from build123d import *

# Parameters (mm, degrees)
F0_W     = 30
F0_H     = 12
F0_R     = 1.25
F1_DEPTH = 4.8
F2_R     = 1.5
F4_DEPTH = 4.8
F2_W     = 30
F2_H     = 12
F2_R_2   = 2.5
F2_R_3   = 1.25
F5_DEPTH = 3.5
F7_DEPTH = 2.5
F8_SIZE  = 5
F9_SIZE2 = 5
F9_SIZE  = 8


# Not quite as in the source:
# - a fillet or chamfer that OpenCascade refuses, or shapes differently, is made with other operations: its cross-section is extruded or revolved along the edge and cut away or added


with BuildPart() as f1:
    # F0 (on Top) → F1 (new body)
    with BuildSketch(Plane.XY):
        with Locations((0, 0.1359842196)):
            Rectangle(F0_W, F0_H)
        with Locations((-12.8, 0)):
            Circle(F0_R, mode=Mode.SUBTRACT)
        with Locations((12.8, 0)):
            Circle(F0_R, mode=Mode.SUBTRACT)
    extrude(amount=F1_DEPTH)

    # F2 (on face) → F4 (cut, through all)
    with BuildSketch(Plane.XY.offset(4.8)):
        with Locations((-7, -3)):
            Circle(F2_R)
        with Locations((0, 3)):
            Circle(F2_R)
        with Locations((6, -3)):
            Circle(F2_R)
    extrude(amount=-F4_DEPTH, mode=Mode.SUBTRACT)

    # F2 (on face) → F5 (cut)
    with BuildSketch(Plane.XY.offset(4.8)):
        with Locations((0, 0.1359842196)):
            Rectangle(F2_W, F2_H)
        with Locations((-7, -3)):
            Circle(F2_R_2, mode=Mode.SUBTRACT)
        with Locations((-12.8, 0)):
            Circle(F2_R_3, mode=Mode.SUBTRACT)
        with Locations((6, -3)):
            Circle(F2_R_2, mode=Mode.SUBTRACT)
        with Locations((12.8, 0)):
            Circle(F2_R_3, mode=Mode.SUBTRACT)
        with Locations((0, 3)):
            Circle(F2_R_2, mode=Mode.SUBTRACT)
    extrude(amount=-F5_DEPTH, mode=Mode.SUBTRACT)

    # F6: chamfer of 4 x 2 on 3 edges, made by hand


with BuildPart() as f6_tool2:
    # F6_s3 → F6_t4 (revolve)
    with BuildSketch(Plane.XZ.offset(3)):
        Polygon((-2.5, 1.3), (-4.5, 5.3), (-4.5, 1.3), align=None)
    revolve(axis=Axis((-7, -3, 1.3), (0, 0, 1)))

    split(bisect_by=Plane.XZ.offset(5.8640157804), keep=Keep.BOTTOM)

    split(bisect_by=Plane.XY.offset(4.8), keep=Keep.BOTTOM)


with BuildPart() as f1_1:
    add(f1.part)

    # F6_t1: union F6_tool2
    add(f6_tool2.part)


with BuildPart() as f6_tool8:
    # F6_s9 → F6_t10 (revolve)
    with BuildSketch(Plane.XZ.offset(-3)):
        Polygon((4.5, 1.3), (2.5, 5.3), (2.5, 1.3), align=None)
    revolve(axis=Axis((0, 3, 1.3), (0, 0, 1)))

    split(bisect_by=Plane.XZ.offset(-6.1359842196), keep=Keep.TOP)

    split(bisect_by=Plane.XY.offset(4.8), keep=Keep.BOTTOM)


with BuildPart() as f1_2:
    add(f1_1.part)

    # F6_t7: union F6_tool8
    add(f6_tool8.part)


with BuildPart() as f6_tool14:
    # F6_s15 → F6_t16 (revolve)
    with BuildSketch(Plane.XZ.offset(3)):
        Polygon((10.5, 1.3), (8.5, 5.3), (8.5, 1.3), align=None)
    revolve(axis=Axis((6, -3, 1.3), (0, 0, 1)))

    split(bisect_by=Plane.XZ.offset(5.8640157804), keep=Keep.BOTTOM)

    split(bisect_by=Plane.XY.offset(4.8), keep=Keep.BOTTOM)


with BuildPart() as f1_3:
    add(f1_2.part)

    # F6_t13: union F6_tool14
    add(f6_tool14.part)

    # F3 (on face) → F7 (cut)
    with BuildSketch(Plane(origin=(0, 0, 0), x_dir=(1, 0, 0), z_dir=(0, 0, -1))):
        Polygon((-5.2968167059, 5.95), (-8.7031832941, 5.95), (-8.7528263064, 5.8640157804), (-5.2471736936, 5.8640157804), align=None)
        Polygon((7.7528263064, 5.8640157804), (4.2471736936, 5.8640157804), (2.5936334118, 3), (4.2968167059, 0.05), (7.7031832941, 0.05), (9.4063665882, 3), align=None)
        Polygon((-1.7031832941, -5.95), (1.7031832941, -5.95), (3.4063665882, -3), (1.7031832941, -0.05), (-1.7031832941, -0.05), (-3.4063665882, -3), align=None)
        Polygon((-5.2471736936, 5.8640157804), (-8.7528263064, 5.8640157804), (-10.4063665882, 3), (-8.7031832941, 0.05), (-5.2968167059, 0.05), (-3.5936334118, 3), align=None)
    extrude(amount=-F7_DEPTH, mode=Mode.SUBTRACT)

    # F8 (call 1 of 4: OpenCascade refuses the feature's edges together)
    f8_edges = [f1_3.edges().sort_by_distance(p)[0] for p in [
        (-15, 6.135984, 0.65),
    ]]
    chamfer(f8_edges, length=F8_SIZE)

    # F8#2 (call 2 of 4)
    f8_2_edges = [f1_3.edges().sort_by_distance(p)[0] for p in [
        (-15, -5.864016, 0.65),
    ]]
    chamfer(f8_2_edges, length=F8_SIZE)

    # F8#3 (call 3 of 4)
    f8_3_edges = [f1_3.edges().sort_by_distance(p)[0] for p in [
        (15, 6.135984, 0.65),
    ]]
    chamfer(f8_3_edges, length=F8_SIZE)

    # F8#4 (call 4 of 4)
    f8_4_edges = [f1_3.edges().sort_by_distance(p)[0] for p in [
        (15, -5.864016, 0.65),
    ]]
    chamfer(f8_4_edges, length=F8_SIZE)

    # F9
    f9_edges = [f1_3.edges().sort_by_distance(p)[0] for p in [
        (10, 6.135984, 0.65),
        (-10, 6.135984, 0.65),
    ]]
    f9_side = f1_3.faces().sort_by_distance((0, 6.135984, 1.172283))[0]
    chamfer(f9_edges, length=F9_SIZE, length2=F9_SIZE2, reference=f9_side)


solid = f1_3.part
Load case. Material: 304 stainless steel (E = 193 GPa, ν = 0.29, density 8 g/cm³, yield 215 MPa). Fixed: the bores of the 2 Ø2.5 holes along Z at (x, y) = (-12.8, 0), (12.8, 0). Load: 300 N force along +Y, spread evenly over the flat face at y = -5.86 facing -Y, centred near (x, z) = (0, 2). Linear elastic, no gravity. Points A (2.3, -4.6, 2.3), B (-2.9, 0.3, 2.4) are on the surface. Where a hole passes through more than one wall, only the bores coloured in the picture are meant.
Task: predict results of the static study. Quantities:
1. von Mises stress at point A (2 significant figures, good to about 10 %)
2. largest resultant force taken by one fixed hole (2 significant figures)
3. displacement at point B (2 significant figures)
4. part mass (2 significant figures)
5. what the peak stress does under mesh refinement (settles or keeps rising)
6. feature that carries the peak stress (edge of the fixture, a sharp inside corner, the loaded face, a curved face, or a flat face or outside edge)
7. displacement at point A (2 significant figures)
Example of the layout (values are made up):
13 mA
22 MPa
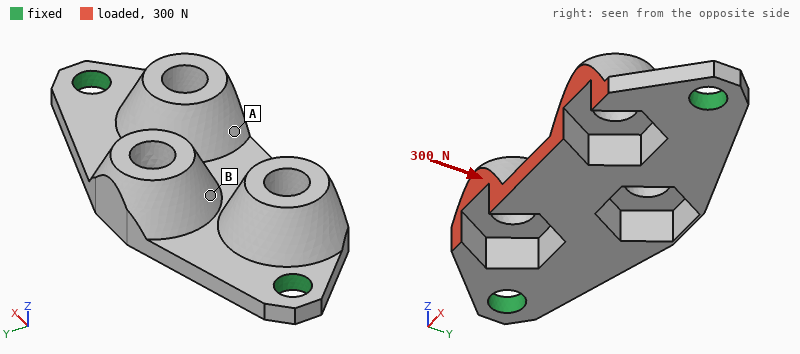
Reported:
30 MPa
150 N
6.7 µm
4.0 g
keeps rising
edge of the fixture
8.2 µm
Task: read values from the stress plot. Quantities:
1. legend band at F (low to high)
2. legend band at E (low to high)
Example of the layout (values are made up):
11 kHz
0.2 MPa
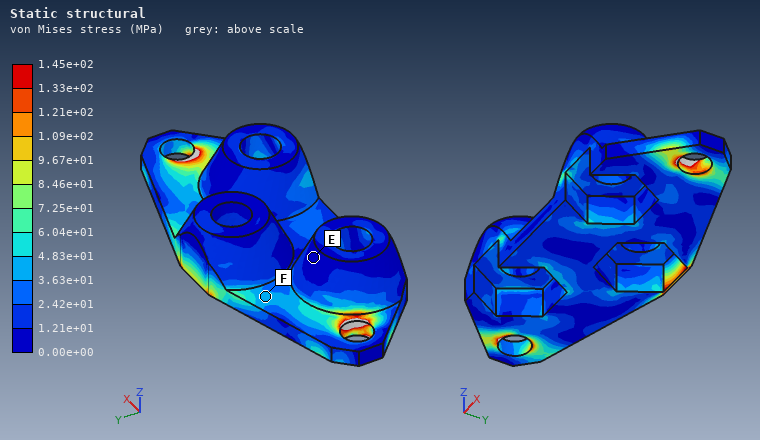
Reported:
3.63e+01 to 4.83e+01 MPa
0.00e+00 to 1.21e+01 MPa
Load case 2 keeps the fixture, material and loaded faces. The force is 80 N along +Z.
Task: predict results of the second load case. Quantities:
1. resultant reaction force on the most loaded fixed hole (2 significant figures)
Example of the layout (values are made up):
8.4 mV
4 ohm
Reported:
72 N
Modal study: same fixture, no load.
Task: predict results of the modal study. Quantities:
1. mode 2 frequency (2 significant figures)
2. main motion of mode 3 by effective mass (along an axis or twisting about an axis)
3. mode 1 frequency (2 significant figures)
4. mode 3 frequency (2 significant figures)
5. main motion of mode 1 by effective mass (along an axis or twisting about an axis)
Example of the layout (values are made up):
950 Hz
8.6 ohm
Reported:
12 kHz
along Y
9900 Hz
22 kHz
along Z
